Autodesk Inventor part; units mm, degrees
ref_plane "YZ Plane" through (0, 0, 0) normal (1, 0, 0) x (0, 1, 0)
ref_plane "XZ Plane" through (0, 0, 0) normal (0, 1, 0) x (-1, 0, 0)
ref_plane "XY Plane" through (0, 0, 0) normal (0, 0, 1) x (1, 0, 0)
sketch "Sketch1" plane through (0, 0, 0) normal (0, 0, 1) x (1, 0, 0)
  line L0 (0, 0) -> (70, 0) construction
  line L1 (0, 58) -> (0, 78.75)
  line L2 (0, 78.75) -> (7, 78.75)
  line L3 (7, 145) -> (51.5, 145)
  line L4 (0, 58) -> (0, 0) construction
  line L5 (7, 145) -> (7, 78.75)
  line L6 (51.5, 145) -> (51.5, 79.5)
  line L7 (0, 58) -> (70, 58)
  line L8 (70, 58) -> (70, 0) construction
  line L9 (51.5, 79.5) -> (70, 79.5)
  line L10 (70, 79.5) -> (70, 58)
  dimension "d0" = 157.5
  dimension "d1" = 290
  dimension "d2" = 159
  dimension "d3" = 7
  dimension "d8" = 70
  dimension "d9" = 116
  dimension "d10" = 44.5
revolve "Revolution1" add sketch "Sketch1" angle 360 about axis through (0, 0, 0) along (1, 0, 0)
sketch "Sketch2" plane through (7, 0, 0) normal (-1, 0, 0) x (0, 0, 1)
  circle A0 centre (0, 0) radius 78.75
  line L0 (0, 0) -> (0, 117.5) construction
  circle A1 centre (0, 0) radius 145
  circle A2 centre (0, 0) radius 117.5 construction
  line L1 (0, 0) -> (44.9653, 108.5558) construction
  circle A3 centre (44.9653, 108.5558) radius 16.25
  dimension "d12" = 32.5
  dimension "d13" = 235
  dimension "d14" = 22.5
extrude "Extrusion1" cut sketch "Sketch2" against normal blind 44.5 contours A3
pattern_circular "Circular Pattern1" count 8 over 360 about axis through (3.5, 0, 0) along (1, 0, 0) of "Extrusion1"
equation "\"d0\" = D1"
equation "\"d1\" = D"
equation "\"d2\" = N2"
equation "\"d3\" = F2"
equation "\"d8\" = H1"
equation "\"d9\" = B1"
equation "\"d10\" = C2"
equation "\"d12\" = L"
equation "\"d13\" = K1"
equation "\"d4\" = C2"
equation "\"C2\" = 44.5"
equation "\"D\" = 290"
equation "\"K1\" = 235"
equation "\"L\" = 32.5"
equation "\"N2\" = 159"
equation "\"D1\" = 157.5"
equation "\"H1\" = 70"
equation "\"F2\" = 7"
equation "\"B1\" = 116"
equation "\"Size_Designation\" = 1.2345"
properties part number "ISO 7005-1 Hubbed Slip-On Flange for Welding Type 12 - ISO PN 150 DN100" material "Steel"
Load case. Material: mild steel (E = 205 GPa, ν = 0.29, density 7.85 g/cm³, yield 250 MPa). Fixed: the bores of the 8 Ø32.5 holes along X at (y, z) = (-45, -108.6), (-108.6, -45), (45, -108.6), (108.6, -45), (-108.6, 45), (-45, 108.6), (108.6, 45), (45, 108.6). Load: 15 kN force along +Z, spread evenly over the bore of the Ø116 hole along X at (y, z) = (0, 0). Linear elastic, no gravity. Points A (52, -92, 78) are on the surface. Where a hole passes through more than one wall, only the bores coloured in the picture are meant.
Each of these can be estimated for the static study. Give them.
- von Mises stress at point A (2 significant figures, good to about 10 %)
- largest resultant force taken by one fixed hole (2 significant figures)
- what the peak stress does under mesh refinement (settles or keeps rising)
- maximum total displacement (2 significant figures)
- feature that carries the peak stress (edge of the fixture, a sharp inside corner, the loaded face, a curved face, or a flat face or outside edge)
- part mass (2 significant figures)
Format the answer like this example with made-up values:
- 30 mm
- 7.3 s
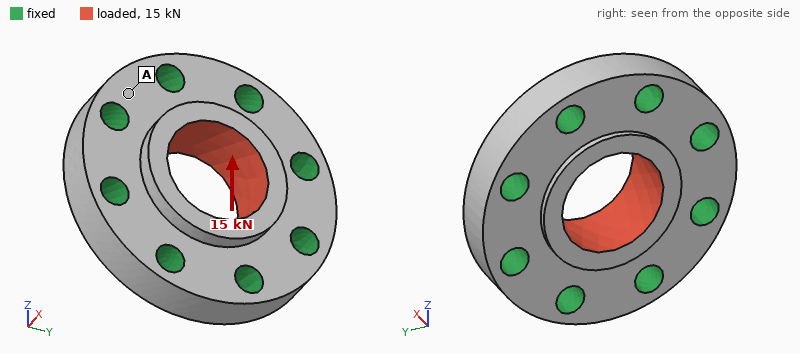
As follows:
- 0.24 MPa
- 2.7 kN
- keeps rising
- 0.54 µm
- edge of the fixture
- 19 kg
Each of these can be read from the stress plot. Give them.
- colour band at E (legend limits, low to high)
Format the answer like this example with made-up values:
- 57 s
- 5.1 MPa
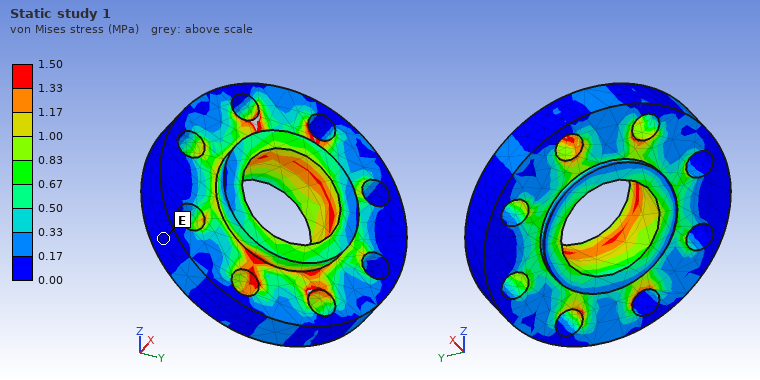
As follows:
- 0.00 to 0.17 MPa
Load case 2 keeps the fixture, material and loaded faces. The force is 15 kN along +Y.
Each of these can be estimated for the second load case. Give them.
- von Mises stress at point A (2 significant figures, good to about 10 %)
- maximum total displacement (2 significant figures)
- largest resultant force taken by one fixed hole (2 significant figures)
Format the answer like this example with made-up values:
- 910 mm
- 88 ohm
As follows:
- 0.26 MPa
- 0.54 µm
- 2.7 kN
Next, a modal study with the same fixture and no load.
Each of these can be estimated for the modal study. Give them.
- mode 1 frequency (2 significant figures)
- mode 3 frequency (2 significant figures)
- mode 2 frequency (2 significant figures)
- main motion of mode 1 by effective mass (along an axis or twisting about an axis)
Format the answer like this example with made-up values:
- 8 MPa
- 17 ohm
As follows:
- 9600 Hz
- 11 kHz
- 11 kHz
- along X
